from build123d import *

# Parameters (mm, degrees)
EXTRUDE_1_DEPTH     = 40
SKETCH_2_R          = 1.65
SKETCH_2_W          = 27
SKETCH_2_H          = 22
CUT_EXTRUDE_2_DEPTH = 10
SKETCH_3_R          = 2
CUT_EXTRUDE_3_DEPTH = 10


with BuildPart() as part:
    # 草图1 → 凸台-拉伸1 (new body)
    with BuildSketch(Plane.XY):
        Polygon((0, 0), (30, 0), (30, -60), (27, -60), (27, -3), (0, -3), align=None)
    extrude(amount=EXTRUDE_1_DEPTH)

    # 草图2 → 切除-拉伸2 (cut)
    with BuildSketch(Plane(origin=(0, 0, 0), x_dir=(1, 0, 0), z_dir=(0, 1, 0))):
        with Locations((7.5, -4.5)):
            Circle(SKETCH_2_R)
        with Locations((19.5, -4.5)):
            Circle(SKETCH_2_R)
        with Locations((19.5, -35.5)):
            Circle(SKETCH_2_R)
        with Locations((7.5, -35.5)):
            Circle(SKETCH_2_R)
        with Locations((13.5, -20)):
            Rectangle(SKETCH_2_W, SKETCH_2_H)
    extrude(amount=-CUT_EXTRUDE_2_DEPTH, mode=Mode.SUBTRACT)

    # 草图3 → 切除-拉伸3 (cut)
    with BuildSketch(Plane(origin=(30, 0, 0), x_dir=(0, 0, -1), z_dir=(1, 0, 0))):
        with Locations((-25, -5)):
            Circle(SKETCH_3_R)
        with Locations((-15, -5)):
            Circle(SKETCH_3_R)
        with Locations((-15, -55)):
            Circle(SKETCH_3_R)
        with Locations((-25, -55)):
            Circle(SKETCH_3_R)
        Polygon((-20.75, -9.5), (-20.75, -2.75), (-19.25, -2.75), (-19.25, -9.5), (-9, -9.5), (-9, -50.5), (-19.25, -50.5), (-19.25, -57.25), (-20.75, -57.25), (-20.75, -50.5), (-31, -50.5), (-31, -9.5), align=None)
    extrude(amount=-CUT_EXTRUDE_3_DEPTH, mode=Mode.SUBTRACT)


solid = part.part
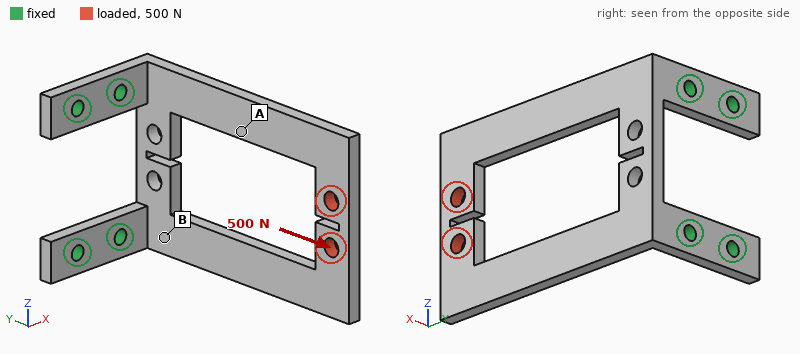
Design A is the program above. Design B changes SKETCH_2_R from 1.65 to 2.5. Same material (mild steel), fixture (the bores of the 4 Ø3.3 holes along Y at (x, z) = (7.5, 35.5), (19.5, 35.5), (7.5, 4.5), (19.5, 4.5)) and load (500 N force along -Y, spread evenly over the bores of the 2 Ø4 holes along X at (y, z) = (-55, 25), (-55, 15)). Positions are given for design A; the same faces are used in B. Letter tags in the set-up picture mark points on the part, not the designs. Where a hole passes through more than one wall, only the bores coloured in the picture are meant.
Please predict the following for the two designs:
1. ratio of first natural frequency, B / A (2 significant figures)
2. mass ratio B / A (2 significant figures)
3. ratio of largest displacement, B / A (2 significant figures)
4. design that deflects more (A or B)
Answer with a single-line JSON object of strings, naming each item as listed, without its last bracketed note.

{"ratio of first natural frequency, B / A": "1.0", "mass ratio B / A": "0.98", "ratio of largest displacement, B / A": "0.77", "design that deflects more": "A"}
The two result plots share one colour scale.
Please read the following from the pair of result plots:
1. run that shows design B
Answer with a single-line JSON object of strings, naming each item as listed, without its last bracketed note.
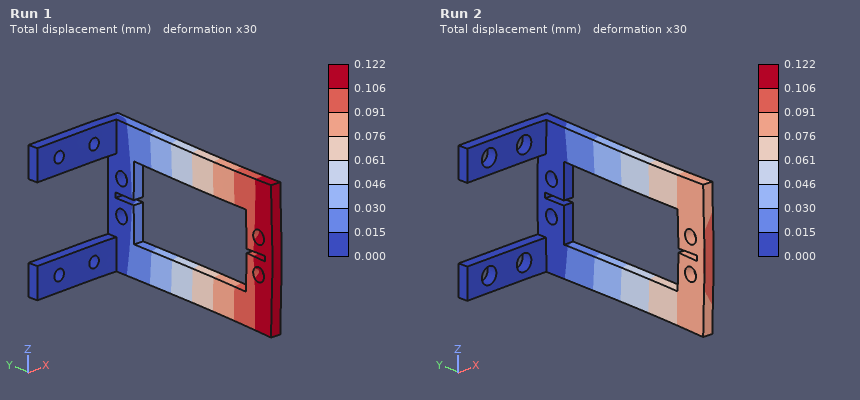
{"run that shows design B": "Run 2"}
